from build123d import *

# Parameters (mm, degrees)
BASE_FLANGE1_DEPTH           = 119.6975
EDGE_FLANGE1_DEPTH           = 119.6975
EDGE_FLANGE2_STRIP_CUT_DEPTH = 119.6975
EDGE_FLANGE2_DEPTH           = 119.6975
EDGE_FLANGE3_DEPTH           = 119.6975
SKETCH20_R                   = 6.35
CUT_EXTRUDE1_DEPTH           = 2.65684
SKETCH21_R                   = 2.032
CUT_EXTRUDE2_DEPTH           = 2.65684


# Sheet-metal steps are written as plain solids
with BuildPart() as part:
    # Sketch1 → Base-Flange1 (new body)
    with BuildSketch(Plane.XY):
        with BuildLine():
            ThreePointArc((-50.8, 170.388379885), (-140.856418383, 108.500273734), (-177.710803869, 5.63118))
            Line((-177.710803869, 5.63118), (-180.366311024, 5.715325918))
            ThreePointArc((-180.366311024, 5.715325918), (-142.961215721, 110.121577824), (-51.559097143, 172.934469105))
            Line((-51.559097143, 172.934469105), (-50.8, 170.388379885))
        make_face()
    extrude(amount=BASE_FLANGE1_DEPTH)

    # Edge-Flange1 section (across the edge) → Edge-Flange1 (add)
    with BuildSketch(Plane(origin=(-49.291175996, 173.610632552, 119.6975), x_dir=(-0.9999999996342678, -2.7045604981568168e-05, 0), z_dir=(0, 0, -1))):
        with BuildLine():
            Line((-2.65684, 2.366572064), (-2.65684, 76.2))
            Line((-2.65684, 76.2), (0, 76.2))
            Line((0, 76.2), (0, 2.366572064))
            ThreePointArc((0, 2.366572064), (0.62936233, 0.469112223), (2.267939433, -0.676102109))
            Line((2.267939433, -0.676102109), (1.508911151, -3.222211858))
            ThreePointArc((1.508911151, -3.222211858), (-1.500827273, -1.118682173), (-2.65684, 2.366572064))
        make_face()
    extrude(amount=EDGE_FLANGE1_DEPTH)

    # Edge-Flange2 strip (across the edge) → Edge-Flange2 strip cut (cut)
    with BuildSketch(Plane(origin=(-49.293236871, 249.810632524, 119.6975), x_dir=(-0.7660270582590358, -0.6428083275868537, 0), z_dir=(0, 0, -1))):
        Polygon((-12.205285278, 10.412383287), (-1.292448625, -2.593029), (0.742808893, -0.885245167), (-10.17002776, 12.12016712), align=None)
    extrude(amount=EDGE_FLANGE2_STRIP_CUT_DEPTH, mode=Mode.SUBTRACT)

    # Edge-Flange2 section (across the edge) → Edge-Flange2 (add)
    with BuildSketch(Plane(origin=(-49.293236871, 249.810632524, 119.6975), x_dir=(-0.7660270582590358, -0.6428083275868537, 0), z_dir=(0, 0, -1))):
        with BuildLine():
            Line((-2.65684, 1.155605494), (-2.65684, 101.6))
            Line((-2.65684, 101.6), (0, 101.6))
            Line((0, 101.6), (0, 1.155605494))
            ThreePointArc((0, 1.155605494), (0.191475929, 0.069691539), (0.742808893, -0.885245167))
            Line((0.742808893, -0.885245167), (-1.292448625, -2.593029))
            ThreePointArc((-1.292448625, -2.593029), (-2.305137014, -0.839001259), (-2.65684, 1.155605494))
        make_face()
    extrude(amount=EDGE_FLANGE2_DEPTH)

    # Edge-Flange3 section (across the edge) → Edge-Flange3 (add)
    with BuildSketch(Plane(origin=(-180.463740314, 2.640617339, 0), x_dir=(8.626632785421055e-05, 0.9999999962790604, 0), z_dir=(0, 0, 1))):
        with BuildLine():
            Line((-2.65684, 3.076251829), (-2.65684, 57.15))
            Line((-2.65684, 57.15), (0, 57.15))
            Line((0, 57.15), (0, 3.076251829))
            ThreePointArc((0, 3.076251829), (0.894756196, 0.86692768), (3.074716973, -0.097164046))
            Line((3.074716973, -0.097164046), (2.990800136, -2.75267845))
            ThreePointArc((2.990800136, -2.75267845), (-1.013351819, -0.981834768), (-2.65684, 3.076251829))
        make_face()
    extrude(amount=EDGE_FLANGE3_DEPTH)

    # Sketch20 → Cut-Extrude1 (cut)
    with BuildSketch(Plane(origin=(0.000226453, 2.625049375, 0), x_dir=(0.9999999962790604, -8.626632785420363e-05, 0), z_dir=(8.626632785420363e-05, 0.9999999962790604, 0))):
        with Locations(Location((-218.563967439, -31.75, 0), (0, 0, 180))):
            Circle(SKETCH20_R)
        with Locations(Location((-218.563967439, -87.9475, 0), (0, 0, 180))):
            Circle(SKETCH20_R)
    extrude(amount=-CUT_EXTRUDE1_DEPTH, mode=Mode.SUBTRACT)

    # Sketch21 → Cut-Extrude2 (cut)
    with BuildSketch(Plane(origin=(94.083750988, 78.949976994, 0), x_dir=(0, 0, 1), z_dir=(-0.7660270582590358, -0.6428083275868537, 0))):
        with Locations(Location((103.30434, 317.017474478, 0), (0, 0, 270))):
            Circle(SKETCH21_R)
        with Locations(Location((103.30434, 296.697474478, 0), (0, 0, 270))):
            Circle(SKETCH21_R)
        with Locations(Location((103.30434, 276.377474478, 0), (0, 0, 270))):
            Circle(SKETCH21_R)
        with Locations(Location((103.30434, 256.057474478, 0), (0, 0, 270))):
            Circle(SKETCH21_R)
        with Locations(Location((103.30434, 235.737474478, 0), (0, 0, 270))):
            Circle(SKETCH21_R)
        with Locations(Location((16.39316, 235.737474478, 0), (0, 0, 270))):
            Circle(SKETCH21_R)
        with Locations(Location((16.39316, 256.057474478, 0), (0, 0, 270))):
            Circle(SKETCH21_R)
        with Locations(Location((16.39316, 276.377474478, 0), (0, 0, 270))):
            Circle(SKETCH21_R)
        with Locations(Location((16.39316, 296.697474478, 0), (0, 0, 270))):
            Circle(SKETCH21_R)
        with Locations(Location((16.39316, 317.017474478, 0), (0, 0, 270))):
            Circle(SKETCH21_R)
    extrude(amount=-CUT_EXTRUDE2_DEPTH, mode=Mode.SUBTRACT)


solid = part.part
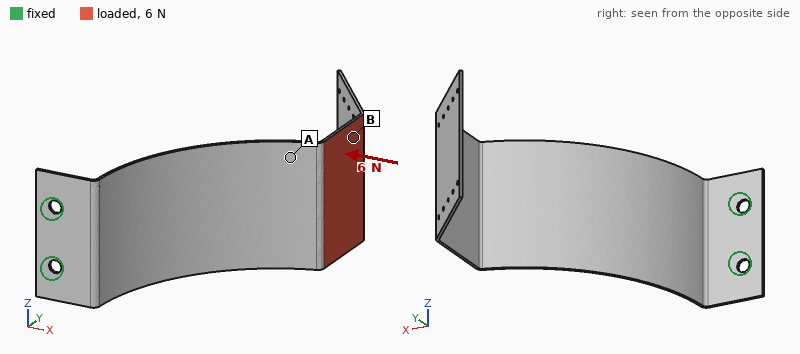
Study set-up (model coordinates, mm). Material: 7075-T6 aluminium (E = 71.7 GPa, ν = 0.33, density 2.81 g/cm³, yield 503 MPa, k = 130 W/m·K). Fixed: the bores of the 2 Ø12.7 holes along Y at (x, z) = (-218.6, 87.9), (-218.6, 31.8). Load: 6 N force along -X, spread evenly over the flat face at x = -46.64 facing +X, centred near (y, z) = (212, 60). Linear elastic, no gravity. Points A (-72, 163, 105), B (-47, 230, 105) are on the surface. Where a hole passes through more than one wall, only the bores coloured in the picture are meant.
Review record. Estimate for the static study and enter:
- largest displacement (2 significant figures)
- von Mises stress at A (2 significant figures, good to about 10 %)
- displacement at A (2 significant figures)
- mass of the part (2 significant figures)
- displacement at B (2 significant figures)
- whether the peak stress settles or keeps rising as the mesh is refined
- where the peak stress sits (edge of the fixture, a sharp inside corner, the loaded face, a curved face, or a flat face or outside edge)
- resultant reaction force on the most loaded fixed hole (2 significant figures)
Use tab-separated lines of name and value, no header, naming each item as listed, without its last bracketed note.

largest displacement	3.8 mm
von Mises stress at A	1.9 MPa
displacement at A	1.8 mm
mass of the part	410 g
displacement at B	2.8 mm
whether the peak stress settles or keeps rising as the mesh is refined	keeps rising
where the peak stress sits	edge of the fixture
resultant reaction force on the most loaded fixed hole	3.7 N
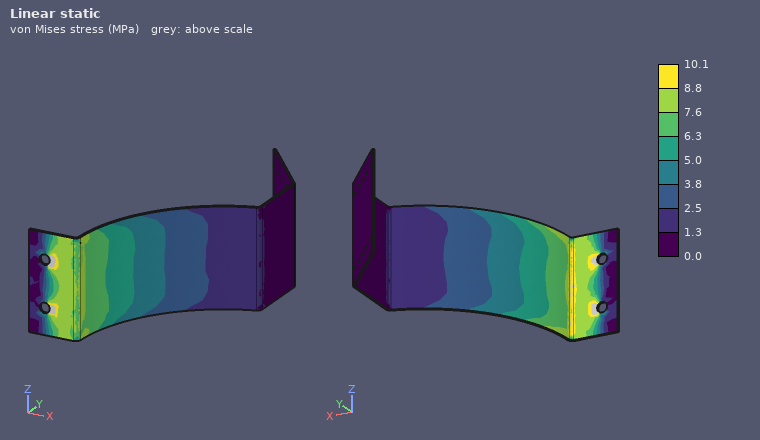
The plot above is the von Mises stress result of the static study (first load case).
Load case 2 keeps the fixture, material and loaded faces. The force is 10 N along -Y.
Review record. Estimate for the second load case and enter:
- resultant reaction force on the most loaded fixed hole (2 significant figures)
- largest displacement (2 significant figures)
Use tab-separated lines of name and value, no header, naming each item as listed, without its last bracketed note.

resultant reaction force on the most loaded fixed hole	5.6 N
largest displacement	4.7 mm
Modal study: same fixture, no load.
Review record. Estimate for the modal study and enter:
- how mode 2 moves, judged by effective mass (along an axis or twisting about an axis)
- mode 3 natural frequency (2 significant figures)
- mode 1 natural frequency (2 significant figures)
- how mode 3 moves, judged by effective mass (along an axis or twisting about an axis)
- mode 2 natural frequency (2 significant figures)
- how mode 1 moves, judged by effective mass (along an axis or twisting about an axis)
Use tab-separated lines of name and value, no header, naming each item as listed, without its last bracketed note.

how mode 2 moves, judged by effective mass	along Z
mode 3 natural frequency	66 Hz
mode 1 natural frequency	13 Hz
how mode 3 moves, judged by effective mass	along Y
mode 2 natural frequency	47 Hz
how mode 1 moves, judged by effective mass	along X
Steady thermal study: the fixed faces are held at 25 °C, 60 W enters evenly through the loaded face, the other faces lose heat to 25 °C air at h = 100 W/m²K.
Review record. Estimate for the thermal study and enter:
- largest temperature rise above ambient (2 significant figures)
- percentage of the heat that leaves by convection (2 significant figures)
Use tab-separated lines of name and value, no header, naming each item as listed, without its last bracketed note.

largest temperature rise above ambient	27 K
percentage of the heat that leaves by convection	100 %
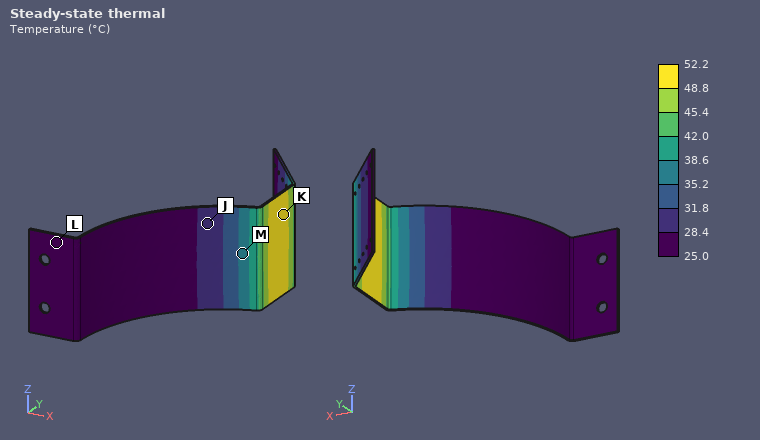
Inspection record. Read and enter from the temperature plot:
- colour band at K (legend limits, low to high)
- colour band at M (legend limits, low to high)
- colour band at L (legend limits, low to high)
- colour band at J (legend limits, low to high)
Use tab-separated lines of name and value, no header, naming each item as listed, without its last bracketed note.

colour band at K	48.8 to 52.2 °C
colour band at M	35.2 to 38.6 °C
colour band at L	25.0 to 28.4 °C
colour band at J	28.4 to 31.8 °C
